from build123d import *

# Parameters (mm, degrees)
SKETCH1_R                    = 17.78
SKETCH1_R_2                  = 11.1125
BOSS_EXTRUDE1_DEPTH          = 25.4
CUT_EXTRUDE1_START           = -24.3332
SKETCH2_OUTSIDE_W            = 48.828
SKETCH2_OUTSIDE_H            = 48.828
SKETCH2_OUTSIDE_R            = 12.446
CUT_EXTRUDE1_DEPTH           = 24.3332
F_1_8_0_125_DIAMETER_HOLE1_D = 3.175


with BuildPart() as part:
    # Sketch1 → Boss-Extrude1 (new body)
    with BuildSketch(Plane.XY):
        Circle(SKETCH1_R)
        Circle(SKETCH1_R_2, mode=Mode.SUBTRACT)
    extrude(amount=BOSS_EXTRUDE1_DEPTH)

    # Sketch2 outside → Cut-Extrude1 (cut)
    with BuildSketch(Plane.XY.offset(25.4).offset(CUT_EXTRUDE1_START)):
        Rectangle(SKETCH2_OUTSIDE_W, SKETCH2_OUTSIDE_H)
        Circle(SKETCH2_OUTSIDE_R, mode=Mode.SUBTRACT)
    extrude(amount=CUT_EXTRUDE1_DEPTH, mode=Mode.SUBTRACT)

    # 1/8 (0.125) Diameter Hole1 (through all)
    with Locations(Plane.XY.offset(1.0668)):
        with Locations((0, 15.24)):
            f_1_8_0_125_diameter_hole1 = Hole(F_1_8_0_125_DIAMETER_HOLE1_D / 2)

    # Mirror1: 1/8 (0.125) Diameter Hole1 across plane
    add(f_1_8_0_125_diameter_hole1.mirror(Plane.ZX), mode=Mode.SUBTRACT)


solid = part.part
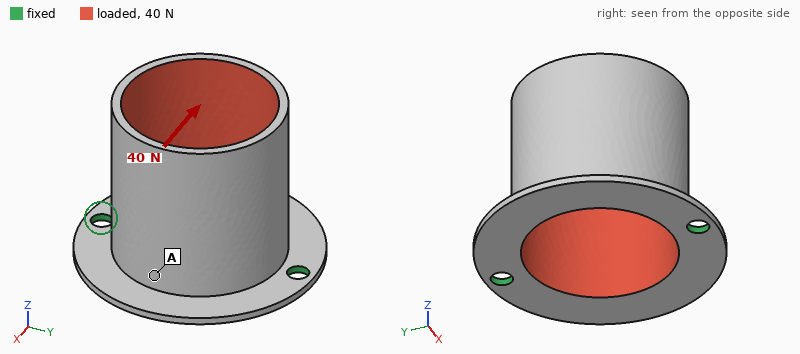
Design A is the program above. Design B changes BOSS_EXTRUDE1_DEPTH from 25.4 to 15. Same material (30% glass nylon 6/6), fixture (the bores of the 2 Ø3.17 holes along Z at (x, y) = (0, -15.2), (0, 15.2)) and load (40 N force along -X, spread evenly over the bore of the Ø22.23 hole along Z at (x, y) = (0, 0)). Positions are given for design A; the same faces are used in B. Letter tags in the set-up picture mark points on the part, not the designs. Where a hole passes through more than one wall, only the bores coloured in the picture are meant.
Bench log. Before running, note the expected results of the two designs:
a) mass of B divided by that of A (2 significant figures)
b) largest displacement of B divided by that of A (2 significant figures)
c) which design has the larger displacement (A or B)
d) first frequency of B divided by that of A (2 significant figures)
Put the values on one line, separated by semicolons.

0.66; 0.41; A; 1.7
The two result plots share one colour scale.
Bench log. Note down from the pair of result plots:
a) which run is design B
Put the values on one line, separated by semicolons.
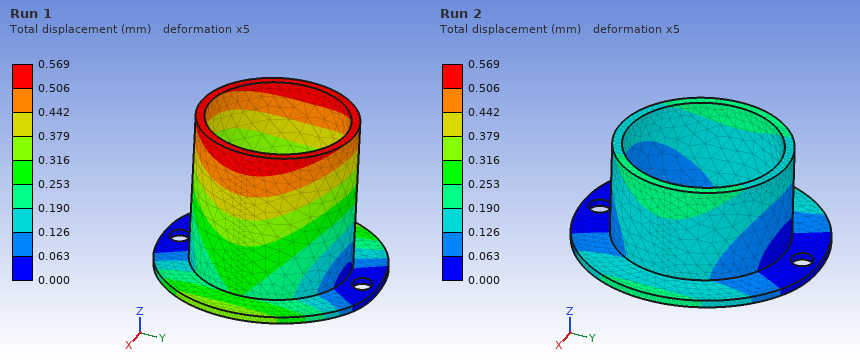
Run 2
